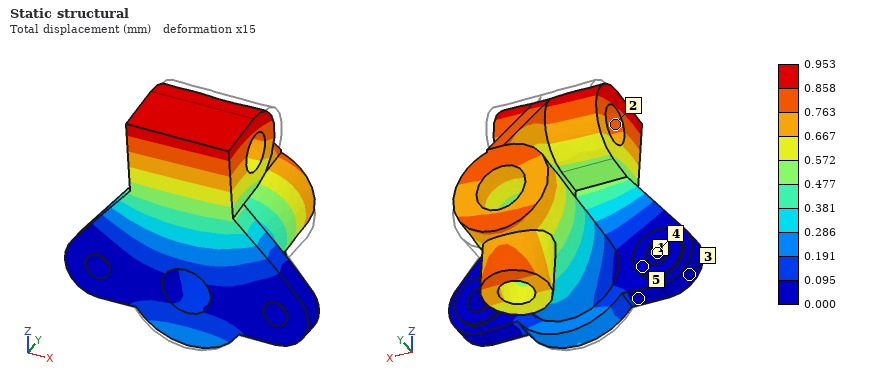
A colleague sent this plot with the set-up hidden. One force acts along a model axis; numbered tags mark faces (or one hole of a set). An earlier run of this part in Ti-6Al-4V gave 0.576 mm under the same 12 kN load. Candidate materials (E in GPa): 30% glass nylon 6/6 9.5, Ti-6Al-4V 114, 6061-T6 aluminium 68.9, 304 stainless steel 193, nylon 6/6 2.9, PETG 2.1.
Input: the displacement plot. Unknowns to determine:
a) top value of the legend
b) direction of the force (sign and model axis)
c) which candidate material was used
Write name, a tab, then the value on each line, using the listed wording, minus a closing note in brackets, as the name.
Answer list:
top value of the legend	0.953 mm
direction of the force	-Y
which candidate material was used	6061-T6 aluminium
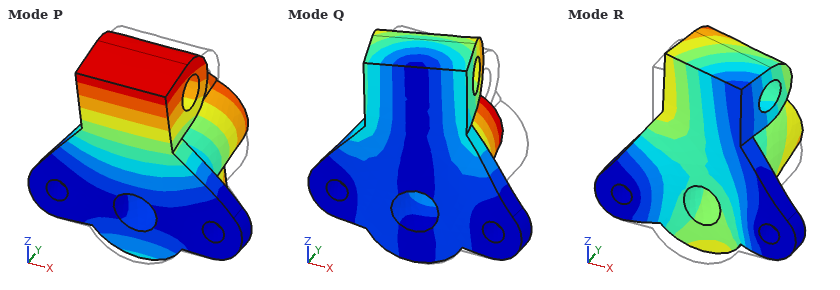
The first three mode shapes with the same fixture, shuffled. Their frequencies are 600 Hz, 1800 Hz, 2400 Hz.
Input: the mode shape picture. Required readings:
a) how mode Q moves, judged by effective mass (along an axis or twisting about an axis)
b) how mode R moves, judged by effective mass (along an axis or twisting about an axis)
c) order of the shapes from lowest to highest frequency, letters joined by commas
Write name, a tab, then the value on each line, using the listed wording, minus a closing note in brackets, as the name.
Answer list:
how mode Q moves, judged by effective mass	along X
how mode R moves, judged by effective mass	along Y
order of the shapes from lowest to highest frequency, letters joined by commas	P, Q, R
